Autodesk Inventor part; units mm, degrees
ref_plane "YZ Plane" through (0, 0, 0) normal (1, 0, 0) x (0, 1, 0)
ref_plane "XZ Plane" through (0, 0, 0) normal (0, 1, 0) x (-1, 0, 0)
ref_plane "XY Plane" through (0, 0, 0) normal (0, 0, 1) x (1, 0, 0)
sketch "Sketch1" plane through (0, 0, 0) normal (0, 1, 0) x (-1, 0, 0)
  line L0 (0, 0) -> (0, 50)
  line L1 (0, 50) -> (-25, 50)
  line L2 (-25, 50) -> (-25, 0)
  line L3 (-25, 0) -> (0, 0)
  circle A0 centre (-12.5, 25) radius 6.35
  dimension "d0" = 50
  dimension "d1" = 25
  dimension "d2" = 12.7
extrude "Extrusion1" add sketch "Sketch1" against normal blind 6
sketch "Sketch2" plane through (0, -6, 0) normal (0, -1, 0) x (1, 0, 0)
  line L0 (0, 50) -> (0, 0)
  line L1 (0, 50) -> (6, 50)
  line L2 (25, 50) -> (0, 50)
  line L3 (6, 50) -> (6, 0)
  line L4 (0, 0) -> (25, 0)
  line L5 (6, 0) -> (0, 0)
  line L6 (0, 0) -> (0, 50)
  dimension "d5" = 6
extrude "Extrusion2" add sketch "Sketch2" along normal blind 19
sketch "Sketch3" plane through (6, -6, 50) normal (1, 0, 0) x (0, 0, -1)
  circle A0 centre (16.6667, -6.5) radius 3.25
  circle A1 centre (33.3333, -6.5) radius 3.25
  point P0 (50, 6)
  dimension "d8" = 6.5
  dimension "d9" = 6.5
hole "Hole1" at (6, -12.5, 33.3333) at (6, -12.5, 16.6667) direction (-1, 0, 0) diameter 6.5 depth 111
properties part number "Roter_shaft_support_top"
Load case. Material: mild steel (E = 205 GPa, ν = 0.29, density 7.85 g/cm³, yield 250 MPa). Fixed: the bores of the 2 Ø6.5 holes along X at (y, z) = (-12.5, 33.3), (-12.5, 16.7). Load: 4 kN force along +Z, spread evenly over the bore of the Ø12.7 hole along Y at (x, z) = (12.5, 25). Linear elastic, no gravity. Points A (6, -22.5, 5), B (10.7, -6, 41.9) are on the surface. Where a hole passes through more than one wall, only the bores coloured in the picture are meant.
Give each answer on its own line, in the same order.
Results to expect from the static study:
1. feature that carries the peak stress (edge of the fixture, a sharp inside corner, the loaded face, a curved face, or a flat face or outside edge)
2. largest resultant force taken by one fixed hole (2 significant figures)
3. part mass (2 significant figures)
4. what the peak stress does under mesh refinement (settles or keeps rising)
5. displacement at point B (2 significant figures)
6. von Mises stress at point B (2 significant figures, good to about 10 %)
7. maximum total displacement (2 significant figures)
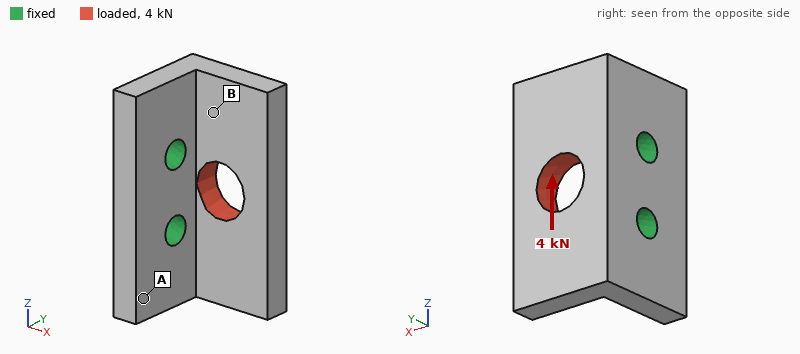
edge of the fixture
2.8 kN
95 g
keeps rising
9.6 µm
30 MPa
22 µm
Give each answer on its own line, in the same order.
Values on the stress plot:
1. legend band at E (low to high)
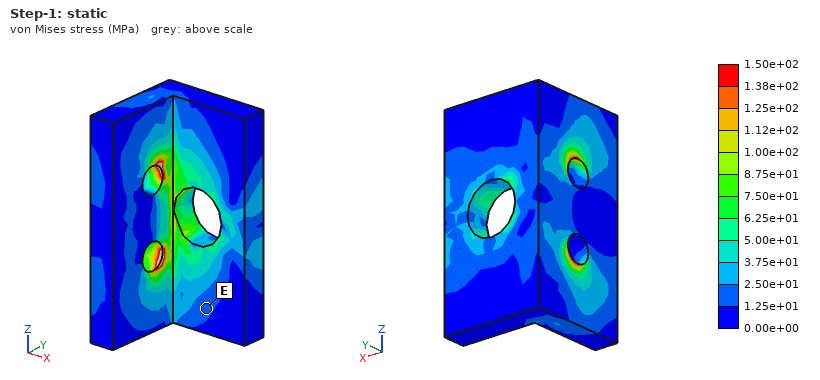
1.25e+01 to 2.50e+01 MPa
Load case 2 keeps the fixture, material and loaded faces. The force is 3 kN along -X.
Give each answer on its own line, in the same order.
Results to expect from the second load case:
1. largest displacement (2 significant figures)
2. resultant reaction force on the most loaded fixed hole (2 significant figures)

18 µm
1.5 kN
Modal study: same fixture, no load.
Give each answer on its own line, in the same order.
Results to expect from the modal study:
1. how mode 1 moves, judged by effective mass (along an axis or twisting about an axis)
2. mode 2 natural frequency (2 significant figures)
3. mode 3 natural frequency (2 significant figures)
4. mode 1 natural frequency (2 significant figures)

along Y
8400 Hz
12 kHz
6300 Hz
